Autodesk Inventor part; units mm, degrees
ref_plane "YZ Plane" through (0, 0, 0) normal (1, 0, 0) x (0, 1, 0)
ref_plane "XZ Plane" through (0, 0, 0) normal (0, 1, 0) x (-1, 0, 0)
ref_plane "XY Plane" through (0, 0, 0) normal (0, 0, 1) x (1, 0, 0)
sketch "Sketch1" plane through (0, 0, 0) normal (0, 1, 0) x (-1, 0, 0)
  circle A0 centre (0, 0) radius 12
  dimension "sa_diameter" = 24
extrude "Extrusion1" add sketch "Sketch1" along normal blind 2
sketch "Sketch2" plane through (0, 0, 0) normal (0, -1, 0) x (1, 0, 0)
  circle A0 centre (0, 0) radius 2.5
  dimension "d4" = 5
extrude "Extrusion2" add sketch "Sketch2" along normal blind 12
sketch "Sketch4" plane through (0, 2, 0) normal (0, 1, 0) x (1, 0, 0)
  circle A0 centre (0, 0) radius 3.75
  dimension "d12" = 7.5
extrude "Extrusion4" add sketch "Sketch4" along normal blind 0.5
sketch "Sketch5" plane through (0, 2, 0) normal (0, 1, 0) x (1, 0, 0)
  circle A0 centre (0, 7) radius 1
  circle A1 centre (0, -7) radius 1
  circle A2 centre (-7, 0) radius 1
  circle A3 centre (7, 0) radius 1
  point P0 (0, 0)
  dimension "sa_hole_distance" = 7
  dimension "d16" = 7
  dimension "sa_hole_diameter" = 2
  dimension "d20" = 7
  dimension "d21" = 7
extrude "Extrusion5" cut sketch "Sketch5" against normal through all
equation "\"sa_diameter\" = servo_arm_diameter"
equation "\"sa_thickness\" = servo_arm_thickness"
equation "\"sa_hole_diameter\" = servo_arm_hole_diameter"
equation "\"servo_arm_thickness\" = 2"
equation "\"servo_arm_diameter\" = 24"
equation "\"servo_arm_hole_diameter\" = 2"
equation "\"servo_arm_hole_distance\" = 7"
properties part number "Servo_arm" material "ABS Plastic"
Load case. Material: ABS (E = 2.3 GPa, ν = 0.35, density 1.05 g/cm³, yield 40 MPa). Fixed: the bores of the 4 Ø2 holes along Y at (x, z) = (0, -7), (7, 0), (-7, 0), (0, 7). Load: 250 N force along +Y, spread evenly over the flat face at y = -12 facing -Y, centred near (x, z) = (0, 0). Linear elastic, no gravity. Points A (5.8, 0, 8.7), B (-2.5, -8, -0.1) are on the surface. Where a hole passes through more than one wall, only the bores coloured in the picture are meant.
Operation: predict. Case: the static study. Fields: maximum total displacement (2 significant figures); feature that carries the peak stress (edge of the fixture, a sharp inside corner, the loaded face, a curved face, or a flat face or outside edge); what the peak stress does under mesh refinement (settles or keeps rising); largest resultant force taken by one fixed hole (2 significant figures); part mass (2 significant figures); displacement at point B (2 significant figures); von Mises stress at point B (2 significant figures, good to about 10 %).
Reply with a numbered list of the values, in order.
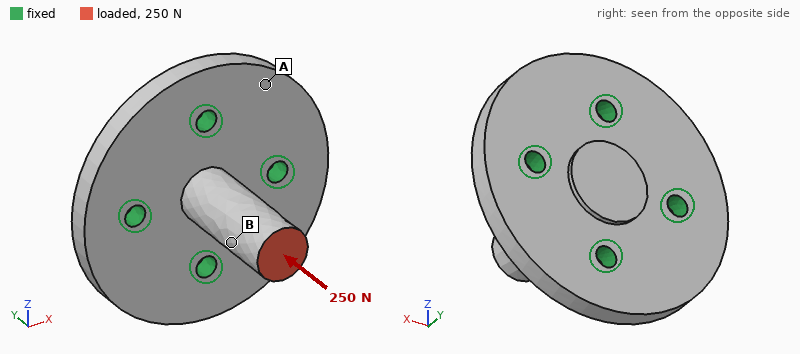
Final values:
1. 0.15 mm
2. edge of the fixture
3. keeps rising
4. 63 N
5. 1.2 g
6. 0.12 mm
7. 13 MPa
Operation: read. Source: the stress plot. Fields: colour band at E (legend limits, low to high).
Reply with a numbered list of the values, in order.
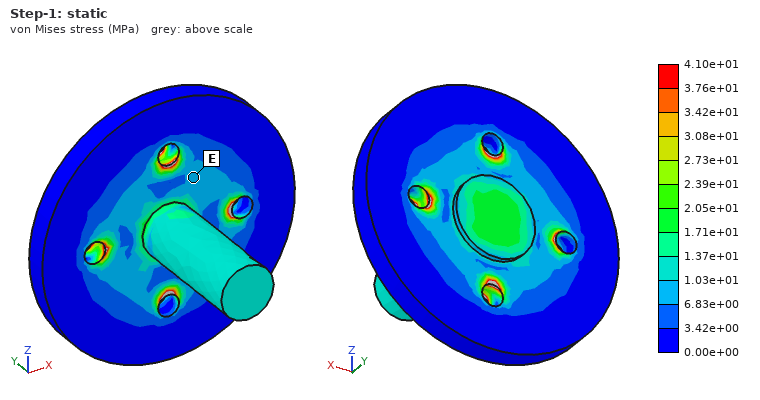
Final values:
1. 6.83e+00 to 1.03e+01 MPa
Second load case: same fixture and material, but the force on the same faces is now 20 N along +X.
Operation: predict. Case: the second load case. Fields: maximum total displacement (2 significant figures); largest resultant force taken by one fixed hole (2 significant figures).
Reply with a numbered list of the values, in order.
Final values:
1. 0.29 mm
2. 23 N
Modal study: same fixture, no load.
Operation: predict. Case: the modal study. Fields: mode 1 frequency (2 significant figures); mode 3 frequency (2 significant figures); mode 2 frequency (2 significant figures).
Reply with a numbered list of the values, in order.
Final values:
1. 4900 Hz
2. 11 kHz
3. 5000 Hz
